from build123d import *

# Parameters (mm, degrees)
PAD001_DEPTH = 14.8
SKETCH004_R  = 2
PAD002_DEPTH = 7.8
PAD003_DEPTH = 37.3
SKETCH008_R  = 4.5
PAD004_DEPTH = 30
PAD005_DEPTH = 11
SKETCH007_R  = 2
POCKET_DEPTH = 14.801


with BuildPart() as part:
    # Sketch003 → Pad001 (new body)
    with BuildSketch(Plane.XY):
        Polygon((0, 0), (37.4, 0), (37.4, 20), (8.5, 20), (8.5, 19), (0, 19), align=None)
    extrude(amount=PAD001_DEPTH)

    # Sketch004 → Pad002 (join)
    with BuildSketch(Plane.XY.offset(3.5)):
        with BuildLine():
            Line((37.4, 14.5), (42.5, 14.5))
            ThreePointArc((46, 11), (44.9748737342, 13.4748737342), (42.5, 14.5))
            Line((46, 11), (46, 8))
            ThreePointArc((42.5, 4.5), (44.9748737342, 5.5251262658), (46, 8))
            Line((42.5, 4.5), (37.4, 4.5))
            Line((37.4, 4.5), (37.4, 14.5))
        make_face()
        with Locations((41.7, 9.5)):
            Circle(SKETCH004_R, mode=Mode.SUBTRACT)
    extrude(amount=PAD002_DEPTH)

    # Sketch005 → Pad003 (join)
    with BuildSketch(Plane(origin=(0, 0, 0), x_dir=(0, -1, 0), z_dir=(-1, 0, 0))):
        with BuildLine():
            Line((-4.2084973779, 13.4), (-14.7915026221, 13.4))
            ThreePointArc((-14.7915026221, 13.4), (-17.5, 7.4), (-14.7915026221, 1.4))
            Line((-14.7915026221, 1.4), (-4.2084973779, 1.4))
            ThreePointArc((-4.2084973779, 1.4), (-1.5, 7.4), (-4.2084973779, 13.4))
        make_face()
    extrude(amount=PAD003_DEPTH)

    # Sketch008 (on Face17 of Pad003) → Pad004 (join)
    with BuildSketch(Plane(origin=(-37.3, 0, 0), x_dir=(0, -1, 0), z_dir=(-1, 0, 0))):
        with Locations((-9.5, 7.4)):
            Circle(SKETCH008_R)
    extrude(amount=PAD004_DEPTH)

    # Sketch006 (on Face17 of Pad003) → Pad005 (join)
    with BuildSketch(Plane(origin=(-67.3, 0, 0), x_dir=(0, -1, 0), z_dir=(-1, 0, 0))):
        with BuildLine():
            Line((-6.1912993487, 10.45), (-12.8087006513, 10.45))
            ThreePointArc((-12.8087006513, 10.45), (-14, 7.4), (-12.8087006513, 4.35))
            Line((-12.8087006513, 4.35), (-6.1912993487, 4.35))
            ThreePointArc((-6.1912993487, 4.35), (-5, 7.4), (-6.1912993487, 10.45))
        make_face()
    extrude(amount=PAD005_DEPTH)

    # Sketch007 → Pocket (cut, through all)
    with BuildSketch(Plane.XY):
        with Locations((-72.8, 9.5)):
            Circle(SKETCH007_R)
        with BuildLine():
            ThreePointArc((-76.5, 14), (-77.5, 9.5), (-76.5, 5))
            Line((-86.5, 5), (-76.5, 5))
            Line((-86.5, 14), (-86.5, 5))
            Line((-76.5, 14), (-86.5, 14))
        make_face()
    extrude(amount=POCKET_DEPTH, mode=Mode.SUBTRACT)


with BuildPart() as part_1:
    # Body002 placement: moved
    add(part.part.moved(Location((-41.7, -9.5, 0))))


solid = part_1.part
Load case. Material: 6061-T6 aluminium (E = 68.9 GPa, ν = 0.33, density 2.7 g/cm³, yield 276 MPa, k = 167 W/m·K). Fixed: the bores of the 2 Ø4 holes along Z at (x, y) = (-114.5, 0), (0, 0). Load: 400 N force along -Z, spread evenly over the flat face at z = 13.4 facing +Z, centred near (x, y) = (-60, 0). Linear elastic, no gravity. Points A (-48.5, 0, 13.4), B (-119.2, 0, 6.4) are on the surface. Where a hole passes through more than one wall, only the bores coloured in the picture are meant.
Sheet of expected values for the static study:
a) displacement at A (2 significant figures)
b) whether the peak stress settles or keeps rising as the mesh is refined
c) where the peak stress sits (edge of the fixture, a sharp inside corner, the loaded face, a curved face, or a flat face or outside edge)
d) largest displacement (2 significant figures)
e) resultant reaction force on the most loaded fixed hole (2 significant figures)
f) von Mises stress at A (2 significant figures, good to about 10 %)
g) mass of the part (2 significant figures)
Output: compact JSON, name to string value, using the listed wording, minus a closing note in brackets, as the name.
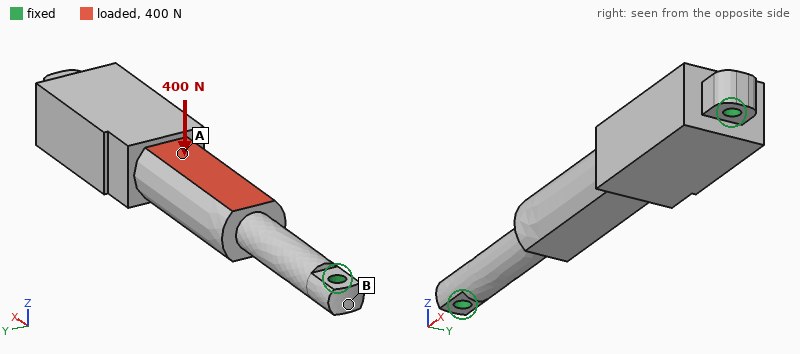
{"displacement at A": "48 µm", "whether the peak stress settles or keeps rising as the mesh is refined": "keeps rising", "where the peak stress sits": "edge of the fixture", "largest displacement": "56 µm", "resultant reaction force on the most loaded fixed hole": "210 N", "von Mises stress at A": "13 MPa", "mass of the part": "55 g"}
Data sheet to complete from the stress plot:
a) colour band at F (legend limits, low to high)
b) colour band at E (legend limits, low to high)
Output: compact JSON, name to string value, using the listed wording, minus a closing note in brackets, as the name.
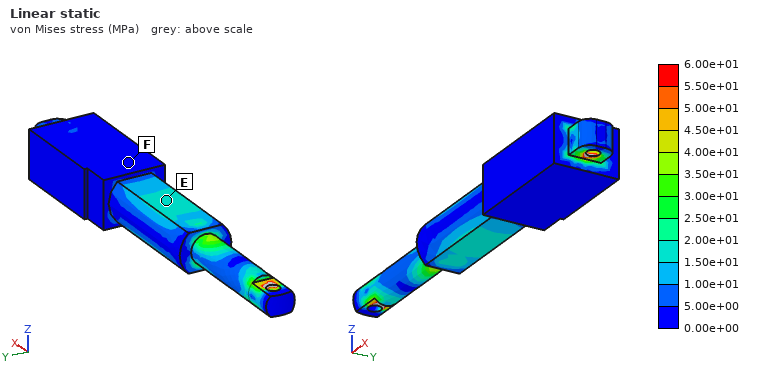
{"colour band at F": "0.00e+00 to 5.00e+00 MPa", "colour band at E": "1.50e+01 to 2.00e+01 MPa"}
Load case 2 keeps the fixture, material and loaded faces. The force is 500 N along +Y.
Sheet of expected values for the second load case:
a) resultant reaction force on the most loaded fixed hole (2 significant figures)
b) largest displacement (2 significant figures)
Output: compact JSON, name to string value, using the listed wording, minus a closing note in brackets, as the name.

{"resultant reaction force on the most loaded fixed hole": "250 N", "largest displacement": "67 µm"}
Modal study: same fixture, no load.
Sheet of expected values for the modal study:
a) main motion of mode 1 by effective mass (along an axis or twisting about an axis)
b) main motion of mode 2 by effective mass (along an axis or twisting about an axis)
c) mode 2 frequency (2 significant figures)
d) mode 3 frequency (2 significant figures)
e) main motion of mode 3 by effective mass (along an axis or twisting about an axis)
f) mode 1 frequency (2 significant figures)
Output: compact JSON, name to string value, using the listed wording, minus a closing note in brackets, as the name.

{"main motion of mode 1 by effective mass": "along Z", "main motion of mode 2 by effective mass": "along Y", "mode 2 frequency": "2900 Hz", "mode 3 frequency": "7400 Hz", "main motion of mode 3 by effective mass": "twisting about X", "mode 1 frequency": "2700 Hz"}
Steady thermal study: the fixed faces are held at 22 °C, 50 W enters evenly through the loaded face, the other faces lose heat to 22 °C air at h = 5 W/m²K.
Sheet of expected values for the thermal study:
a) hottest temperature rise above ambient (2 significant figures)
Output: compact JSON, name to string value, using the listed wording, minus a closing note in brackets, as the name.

{"hottest temperature rise above ambient": "58 K"}
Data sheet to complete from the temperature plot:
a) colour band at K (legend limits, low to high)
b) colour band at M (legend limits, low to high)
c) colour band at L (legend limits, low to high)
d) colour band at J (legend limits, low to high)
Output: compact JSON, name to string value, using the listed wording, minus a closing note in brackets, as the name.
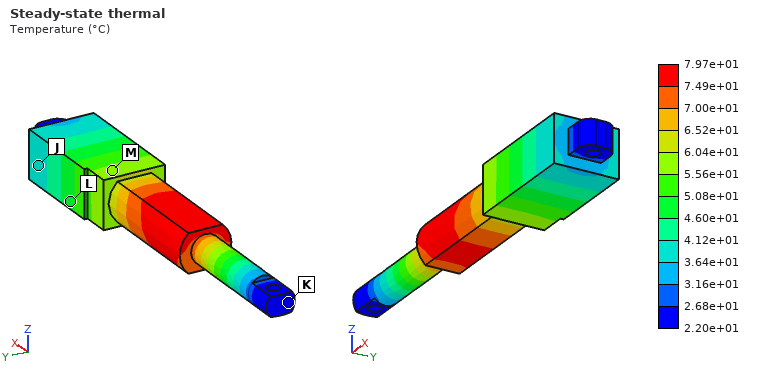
{"colour band at K": "2.20e+01 to 2.68e+01 °C", "colour band at M": "5.56e+01 to 6.04e+01 °C", "colour band at L": "4.60e+01 to 5.08e+01 °C", "colour band at J": "3.64e+01 to 4.12e+01 °C"}
